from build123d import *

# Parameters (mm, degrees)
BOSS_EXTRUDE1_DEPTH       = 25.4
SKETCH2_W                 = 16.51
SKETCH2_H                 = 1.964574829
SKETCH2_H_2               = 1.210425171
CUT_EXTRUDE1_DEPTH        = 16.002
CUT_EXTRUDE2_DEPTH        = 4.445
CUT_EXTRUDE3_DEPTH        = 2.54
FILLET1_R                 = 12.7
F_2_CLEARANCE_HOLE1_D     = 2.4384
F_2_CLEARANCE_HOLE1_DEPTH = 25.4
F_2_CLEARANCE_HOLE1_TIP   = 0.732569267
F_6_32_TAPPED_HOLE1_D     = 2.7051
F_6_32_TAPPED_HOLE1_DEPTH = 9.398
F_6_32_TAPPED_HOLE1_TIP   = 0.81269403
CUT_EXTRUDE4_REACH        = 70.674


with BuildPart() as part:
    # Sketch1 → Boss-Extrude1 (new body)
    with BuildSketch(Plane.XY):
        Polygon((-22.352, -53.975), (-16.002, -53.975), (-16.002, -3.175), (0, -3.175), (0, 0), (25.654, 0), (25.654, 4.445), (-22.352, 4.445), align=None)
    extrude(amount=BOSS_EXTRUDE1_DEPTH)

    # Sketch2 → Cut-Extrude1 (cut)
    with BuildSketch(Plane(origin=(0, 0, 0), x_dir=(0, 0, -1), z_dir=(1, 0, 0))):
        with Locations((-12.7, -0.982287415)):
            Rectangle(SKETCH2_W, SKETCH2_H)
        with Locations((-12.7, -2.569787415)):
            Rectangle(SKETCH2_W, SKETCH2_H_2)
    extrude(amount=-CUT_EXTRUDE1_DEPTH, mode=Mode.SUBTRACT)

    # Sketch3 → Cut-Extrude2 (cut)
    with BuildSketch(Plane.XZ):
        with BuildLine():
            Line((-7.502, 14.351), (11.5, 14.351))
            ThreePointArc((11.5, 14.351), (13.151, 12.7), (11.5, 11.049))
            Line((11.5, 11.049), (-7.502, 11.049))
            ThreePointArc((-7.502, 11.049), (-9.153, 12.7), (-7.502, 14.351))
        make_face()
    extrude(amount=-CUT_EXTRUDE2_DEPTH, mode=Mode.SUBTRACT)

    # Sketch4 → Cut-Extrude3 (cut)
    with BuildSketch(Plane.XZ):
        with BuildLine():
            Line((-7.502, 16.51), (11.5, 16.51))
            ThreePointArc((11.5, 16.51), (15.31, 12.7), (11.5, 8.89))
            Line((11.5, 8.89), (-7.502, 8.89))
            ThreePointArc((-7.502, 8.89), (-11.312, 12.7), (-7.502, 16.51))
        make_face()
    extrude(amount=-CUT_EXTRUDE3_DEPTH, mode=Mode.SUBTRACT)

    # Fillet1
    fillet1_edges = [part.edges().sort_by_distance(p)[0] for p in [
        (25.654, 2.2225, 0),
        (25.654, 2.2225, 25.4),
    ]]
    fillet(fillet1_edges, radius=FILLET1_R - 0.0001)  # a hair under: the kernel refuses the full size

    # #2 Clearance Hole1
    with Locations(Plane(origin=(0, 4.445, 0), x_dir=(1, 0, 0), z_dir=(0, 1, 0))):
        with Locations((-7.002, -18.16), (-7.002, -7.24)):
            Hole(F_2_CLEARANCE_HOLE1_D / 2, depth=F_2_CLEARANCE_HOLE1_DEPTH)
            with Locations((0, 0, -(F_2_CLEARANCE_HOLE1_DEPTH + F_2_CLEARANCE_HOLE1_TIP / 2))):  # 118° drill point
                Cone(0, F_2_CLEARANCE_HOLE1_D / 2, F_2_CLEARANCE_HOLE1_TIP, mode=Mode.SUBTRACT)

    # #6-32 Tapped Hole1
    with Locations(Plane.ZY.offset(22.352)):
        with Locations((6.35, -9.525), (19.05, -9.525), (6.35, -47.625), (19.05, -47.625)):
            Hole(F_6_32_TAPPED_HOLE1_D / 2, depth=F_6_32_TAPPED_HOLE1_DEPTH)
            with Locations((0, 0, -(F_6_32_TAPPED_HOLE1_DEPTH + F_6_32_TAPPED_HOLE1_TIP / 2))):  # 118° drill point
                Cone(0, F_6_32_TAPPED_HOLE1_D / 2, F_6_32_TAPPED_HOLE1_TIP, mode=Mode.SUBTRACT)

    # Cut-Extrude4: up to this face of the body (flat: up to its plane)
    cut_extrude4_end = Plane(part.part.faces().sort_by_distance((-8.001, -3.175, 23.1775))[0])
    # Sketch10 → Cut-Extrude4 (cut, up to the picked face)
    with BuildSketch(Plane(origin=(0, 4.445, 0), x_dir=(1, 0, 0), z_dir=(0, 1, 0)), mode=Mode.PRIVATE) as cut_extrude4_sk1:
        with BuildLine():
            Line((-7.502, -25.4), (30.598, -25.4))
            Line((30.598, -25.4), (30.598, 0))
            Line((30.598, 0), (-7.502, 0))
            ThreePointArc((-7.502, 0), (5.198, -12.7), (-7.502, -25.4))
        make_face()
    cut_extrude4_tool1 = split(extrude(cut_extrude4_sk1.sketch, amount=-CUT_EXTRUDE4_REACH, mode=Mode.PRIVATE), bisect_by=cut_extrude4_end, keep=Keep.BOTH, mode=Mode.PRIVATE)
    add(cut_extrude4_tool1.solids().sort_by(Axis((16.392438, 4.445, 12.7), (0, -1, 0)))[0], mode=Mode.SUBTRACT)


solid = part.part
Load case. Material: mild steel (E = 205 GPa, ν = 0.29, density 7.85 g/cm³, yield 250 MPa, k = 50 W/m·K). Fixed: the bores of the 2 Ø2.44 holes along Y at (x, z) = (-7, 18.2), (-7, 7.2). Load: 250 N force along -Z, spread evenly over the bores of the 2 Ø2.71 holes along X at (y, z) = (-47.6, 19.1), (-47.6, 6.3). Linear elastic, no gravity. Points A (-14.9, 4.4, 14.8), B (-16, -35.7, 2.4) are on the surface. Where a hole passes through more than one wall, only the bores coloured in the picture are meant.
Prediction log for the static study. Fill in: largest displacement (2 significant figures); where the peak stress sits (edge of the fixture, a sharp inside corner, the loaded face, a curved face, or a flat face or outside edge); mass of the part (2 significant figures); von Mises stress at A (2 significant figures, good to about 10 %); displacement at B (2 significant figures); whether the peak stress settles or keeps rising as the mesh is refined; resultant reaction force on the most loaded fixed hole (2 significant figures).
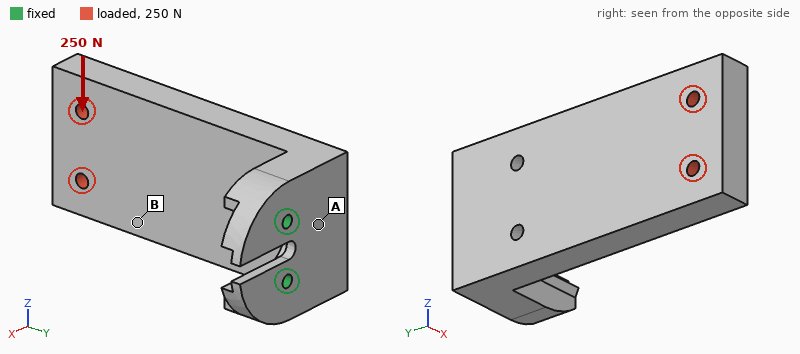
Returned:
63 µm
edge of the fixture
89 g
42 MPa
42 µm
keeps rising
690 N
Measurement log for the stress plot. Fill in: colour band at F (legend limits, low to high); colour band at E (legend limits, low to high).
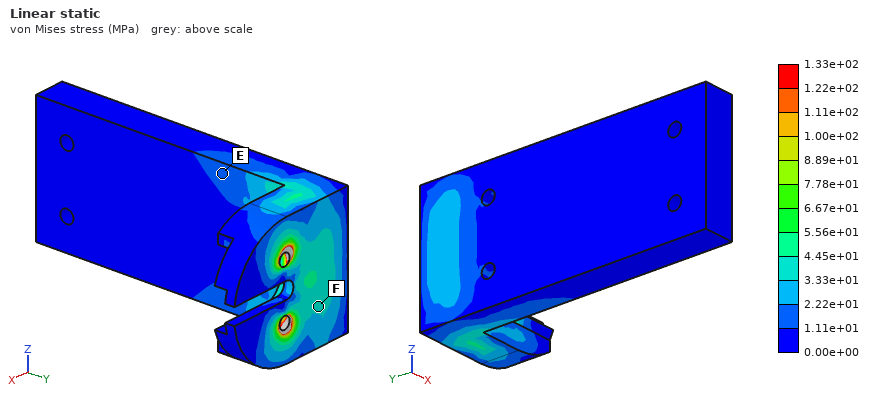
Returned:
3.33e+01 to 4.45e+01 MPa
1.11e+01 to 2.22e+01 MPa
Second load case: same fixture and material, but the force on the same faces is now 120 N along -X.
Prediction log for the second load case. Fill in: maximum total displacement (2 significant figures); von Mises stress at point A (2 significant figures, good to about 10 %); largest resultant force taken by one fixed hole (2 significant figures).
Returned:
0.11 mm
25 MPa
95 N
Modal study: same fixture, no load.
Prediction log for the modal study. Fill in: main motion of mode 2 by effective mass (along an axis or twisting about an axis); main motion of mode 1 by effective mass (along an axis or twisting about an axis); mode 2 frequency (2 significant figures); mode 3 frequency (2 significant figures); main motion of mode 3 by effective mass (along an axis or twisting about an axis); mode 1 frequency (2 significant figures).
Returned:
along Z
along X
2000 Hz
5700 Hz
along Y
1100 Hz
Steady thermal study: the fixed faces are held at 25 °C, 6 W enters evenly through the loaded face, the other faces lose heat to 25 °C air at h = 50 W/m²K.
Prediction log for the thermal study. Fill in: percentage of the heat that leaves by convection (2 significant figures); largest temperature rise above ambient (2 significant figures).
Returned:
56 %
29 K
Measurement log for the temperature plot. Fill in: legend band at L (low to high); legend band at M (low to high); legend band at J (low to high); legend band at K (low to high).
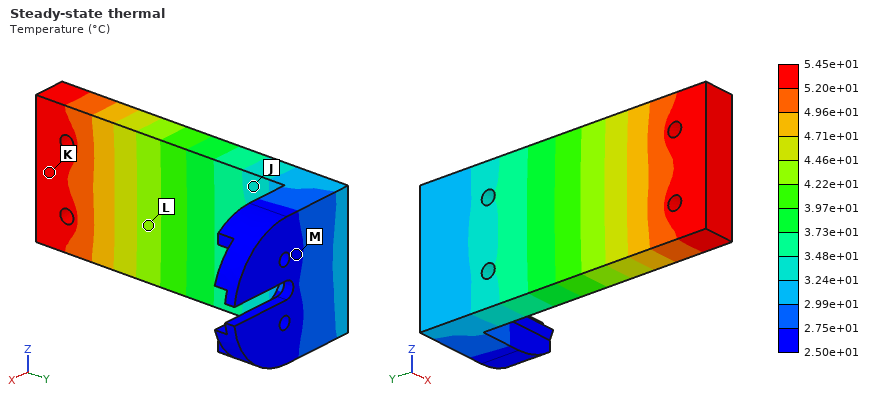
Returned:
4.22e+01 to 4.46e+01 °C
2.50e+01 to 2.75e+01 °C
3.24e+01 to 3.48e+01 °C
5.20e+01 to 5.45e+01 °C
